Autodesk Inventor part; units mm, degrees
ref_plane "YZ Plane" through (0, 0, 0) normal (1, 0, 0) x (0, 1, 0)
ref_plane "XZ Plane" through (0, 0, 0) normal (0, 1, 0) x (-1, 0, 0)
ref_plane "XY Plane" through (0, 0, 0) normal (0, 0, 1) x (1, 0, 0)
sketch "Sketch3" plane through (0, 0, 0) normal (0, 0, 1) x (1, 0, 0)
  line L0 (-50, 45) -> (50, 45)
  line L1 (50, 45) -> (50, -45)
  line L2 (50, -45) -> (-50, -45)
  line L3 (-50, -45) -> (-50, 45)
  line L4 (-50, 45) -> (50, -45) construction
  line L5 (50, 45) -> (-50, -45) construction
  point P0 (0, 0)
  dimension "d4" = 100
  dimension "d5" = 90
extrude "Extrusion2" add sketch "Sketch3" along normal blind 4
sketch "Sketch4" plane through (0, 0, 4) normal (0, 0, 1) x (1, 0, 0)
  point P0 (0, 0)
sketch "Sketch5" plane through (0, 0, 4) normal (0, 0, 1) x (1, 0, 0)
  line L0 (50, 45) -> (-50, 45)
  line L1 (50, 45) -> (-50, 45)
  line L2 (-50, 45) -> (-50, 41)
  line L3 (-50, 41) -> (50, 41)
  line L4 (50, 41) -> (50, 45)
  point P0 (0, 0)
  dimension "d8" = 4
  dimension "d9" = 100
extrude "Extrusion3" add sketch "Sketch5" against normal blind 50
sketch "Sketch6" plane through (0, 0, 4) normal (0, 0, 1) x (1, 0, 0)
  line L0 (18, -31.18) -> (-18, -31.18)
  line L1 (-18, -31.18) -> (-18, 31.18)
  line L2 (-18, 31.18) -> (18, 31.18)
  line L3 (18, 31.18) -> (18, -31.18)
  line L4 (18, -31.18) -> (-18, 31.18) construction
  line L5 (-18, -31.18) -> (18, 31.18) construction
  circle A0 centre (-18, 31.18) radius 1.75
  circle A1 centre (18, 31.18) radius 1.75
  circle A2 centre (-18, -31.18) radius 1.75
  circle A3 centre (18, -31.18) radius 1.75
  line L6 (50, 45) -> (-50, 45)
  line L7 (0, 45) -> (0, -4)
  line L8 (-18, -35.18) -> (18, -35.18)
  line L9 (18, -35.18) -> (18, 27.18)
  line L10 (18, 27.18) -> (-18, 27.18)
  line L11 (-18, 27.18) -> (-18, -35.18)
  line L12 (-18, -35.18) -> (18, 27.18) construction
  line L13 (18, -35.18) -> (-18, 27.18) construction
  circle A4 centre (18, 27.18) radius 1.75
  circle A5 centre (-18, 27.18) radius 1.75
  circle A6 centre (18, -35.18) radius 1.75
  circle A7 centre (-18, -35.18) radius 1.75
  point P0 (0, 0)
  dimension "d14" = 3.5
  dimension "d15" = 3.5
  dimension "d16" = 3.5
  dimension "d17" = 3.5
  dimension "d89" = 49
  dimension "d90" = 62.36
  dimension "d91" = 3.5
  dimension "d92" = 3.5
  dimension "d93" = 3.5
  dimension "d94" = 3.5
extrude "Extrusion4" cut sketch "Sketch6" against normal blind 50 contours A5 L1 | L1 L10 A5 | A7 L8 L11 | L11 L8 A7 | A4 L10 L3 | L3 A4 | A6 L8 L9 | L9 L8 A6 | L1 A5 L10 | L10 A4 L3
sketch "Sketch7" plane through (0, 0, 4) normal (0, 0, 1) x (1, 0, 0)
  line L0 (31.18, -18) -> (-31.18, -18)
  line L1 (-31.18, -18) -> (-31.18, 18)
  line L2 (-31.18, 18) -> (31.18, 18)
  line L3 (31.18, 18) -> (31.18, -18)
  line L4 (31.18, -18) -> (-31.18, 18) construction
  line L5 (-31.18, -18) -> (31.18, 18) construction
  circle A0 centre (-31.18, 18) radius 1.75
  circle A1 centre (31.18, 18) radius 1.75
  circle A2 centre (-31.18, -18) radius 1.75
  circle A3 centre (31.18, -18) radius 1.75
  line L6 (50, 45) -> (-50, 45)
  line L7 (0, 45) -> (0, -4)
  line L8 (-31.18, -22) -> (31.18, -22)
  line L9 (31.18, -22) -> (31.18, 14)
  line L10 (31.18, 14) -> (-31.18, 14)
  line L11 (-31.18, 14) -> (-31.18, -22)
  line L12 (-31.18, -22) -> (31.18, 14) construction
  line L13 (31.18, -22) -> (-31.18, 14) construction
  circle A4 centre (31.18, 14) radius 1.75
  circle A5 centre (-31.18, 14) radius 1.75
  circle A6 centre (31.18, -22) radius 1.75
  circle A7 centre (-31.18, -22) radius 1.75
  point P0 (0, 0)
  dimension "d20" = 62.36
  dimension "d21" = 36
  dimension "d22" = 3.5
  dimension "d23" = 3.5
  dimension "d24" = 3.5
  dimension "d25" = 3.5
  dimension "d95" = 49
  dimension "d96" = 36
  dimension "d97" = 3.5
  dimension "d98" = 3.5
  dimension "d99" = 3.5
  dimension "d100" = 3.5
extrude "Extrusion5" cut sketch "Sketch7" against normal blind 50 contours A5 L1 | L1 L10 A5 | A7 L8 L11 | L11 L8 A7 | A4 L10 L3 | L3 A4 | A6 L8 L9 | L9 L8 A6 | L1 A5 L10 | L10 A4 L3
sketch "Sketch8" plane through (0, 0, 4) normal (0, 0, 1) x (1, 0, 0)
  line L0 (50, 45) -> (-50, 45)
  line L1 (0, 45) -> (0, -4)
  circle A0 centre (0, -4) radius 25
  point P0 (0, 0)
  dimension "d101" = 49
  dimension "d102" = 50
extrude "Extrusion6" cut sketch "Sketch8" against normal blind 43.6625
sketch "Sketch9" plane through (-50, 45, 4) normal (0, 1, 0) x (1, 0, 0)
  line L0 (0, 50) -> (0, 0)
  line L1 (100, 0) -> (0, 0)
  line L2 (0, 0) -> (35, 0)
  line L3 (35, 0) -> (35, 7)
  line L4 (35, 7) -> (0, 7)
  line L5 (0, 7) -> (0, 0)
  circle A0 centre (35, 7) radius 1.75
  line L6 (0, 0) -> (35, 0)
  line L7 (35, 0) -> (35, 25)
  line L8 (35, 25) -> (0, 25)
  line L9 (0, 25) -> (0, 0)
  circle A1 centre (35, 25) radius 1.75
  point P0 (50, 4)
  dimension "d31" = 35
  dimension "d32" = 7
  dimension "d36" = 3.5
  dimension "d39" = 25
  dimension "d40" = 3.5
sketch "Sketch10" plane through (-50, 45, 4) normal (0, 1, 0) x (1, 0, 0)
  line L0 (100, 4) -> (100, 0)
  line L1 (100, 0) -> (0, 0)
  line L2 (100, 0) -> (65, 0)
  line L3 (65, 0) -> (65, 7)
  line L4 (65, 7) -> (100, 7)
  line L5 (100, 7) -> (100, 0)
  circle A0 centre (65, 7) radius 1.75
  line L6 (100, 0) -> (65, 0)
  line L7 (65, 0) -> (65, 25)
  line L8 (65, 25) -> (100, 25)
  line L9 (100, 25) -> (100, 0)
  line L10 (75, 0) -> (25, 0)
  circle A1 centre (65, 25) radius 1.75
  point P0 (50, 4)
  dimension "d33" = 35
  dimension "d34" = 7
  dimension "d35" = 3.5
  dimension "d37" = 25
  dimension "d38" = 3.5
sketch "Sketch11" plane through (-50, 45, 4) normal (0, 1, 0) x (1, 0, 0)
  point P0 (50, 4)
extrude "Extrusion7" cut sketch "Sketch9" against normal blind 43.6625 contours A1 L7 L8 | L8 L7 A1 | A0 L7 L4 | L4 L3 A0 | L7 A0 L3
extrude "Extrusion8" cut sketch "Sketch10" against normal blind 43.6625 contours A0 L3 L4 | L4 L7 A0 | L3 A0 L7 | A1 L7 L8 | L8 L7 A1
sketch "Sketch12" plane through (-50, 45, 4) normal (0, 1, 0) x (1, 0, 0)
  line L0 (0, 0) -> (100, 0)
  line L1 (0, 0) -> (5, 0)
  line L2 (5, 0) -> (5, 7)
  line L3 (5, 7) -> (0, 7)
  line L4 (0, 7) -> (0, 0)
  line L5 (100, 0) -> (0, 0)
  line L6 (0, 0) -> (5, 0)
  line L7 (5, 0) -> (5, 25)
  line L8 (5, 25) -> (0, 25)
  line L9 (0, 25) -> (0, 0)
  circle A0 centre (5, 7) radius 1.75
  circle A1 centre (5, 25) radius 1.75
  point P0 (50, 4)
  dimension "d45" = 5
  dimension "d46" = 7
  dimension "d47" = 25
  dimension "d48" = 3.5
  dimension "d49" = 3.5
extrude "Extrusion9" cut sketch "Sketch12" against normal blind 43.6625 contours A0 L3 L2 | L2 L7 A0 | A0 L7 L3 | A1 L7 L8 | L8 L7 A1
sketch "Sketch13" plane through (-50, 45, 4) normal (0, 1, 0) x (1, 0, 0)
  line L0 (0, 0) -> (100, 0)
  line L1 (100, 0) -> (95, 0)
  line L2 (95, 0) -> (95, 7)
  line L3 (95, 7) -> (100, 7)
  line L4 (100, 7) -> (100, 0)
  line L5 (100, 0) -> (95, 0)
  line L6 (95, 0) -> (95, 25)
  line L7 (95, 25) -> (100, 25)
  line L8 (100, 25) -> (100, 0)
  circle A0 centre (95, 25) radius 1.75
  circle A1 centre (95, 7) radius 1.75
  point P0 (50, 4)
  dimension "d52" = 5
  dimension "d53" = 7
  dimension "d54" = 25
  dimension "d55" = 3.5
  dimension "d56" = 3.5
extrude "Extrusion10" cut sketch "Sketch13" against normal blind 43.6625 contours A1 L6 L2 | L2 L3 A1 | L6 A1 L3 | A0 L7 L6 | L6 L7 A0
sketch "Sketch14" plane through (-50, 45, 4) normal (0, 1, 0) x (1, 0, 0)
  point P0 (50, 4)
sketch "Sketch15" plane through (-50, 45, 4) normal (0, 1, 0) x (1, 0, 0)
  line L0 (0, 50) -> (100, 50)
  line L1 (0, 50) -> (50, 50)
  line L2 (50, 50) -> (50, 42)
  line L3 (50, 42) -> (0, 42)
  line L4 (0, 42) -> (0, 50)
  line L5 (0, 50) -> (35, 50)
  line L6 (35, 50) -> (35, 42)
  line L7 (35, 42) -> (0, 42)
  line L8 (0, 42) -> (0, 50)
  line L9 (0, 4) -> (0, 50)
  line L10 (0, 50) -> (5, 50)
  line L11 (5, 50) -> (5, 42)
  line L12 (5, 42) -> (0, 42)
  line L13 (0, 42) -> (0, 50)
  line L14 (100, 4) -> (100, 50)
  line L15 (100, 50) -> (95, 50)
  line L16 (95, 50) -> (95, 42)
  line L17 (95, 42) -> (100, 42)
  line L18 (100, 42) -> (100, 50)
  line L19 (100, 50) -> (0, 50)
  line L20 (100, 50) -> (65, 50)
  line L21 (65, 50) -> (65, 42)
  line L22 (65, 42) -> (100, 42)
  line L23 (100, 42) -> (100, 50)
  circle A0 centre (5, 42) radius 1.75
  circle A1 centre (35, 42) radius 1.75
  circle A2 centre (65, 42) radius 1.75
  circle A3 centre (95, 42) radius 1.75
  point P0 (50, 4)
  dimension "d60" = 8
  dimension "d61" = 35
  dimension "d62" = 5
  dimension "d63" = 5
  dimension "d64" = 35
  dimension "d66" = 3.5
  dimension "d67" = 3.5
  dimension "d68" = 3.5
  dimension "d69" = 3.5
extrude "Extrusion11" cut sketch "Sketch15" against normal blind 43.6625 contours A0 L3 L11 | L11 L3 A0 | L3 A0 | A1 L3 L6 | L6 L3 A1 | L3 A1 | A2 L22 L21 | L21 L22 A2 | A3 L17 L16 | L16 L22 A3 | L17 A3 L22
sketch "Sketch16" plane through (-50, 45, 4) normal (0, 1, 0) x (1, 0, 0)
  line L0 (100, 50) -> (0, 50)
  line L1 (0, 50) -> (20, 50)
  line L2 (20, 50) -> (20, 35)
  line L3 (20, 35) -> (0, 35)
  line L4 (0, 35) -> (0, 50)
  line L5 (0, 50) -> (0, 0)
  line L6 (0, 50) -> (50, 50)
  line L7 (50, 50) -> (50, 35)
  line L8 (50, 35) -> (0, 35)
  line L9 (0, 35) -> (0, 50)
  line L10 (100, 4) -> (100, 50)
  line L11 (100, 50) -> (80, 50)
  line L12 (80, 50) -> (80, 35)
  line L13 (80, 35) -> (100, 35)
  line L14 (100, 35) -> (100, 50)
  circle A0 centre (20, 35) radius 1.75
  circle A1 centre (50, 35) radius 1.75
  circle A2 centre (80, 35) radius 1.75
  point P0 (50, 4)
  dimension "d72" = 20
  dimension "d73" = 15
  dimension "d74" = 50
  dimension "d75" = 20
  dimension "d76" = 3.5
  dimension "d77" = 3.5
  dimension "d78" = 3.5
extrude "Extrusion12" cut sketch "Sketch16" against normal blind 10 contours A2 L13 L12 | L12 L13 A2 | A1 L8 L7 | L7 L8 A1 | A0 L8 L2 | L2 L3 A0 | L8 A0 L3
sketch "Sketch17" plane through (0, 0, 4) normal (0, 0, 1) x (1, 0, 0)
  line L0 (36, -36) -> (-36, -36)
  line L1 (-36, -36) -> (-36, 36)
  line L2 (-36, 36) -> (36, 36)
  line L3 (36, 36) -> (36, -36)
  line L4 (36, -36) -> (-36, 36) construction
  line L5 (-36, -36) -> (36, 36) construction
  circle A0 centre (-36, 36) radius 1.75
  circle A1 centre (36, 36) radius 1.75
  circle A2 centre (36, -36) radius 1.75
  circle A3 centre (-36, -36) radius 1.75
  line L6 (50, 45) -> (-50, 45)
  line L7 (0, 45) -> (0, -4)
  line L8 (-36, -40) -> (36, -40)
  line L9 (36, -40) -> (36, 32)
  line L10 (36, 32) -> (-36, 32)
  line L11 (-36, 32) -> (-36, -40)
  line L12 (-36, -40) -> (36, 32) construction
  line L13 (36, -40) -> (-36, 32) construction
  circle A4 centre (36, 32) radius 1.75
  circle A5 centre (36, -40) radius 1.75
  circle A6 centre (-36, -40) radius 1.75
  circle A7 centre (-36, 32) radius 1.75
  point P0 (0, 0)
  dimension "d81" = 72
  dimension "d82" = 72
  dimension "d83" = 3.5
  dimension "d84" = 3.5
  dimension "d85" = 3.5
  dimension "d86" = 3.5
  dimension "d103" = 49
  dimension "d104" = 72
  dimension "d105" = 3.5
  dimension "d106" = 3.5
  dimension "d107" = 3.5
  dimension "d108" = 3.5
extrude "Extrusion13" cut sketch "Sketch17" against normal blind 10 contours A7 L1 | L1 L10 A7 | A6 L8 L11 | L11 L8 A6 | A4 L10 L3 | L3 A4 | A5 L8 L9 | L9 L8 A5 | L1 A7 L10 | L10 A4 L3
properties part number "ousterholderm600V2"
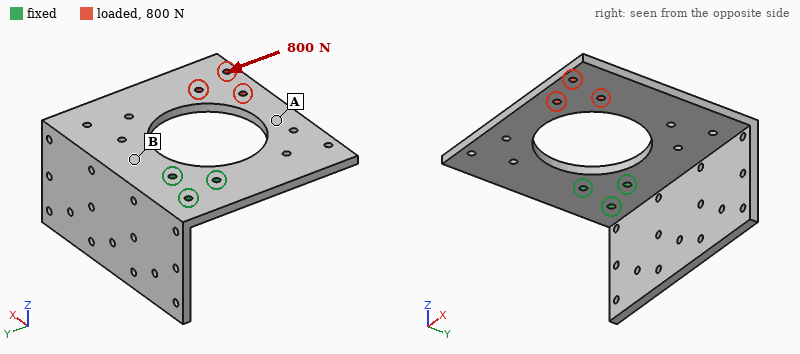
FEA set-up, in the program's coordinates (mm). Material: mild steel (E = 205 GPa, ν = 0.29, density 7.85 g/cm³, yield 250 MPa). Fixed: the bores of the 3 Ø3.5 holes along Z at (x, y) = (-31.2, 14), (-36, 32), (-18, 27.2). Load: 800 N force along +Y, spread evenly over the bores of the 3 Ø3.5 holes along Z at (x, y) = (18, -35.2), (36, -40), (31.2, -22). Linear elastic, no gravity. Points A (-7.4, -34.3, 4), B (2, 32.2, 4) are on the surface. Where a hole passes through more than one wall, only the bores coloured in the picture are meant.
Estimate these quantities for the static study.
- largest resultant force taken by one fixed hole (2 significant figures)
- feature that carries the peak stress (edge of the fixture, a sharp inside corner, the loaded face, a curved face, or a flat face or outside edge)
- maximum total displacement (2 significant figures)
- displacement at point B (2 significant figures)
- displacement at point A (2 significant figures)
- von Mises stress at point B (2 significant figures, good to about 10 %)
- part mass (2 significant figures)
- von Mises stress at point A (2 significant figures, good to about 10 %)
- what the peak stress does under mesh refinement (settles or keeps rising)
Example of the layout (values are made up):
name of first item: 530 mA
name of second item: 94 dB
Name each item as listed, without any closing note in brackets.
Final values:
largest resultant force taken by one fixed hole: 1.5 kN
feature that carries the peak stress: edge of the fixture
maximum total displacement: 34 µm
displacement at point B: 7.5 µm
displacement at point A: 20 µm
von Mises stress at point B: 17 MPa
part mass: 360 g
von Mises stress at point A: 6.4 MPa
what the peak stress does under mesh refinement: keeps rising
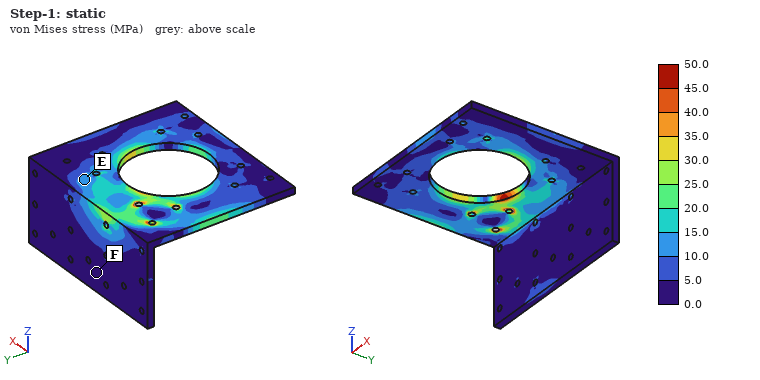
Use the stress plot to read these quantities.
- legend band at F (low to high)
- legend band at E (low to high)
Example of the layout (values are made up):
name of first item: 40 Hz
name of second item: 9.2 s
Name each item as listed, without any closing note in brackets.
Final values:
legend band at F: 0.0 to 5.0 MPa
legend band at E: 10.0 to 15.0 MPa
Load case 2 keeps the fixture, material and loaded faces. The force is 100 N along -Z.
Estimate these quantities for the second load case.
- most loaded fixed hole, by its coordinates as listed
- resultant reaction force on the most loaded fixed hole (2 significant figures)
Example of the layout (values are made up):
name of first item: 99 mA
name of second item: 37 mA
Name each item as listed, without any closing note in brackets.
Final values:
most loaded fixed hole, by its coordinates as listed: (-36, 32)
resultant reaction force on the most loaded fixed hole: 220 N
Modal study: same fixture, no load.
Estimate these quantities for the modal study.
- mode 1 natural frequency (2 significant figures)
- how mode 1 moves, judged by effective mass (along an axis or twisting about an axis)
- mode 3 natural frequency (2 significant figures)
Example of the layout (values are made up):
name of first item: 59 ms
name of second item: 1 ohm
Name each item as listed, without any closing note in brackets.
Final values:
mode 1 natural frequency: 440 Hz
how mode 1 moves, judged by effective mass: along Z
mode 3 natural frequency: 920 Hz
